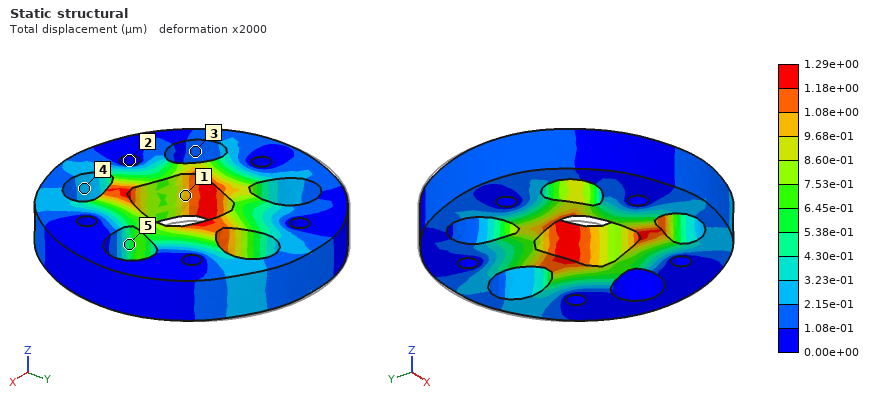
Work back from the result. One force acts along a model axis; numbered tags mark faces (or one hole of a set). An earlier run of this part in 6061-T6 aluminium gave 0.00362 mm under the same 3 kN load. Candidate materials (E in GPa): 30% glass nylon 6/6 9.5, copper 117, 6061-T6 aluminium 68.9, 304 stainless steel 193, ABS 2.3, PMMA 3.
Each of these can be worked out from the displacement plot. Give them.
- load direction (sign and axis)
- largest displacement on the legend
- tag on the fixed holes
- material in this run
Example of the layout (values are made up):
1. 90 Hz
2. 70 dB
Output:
1. -Y
2. 1.29e+00 µm
3. 2
4. 304 stainless steel
